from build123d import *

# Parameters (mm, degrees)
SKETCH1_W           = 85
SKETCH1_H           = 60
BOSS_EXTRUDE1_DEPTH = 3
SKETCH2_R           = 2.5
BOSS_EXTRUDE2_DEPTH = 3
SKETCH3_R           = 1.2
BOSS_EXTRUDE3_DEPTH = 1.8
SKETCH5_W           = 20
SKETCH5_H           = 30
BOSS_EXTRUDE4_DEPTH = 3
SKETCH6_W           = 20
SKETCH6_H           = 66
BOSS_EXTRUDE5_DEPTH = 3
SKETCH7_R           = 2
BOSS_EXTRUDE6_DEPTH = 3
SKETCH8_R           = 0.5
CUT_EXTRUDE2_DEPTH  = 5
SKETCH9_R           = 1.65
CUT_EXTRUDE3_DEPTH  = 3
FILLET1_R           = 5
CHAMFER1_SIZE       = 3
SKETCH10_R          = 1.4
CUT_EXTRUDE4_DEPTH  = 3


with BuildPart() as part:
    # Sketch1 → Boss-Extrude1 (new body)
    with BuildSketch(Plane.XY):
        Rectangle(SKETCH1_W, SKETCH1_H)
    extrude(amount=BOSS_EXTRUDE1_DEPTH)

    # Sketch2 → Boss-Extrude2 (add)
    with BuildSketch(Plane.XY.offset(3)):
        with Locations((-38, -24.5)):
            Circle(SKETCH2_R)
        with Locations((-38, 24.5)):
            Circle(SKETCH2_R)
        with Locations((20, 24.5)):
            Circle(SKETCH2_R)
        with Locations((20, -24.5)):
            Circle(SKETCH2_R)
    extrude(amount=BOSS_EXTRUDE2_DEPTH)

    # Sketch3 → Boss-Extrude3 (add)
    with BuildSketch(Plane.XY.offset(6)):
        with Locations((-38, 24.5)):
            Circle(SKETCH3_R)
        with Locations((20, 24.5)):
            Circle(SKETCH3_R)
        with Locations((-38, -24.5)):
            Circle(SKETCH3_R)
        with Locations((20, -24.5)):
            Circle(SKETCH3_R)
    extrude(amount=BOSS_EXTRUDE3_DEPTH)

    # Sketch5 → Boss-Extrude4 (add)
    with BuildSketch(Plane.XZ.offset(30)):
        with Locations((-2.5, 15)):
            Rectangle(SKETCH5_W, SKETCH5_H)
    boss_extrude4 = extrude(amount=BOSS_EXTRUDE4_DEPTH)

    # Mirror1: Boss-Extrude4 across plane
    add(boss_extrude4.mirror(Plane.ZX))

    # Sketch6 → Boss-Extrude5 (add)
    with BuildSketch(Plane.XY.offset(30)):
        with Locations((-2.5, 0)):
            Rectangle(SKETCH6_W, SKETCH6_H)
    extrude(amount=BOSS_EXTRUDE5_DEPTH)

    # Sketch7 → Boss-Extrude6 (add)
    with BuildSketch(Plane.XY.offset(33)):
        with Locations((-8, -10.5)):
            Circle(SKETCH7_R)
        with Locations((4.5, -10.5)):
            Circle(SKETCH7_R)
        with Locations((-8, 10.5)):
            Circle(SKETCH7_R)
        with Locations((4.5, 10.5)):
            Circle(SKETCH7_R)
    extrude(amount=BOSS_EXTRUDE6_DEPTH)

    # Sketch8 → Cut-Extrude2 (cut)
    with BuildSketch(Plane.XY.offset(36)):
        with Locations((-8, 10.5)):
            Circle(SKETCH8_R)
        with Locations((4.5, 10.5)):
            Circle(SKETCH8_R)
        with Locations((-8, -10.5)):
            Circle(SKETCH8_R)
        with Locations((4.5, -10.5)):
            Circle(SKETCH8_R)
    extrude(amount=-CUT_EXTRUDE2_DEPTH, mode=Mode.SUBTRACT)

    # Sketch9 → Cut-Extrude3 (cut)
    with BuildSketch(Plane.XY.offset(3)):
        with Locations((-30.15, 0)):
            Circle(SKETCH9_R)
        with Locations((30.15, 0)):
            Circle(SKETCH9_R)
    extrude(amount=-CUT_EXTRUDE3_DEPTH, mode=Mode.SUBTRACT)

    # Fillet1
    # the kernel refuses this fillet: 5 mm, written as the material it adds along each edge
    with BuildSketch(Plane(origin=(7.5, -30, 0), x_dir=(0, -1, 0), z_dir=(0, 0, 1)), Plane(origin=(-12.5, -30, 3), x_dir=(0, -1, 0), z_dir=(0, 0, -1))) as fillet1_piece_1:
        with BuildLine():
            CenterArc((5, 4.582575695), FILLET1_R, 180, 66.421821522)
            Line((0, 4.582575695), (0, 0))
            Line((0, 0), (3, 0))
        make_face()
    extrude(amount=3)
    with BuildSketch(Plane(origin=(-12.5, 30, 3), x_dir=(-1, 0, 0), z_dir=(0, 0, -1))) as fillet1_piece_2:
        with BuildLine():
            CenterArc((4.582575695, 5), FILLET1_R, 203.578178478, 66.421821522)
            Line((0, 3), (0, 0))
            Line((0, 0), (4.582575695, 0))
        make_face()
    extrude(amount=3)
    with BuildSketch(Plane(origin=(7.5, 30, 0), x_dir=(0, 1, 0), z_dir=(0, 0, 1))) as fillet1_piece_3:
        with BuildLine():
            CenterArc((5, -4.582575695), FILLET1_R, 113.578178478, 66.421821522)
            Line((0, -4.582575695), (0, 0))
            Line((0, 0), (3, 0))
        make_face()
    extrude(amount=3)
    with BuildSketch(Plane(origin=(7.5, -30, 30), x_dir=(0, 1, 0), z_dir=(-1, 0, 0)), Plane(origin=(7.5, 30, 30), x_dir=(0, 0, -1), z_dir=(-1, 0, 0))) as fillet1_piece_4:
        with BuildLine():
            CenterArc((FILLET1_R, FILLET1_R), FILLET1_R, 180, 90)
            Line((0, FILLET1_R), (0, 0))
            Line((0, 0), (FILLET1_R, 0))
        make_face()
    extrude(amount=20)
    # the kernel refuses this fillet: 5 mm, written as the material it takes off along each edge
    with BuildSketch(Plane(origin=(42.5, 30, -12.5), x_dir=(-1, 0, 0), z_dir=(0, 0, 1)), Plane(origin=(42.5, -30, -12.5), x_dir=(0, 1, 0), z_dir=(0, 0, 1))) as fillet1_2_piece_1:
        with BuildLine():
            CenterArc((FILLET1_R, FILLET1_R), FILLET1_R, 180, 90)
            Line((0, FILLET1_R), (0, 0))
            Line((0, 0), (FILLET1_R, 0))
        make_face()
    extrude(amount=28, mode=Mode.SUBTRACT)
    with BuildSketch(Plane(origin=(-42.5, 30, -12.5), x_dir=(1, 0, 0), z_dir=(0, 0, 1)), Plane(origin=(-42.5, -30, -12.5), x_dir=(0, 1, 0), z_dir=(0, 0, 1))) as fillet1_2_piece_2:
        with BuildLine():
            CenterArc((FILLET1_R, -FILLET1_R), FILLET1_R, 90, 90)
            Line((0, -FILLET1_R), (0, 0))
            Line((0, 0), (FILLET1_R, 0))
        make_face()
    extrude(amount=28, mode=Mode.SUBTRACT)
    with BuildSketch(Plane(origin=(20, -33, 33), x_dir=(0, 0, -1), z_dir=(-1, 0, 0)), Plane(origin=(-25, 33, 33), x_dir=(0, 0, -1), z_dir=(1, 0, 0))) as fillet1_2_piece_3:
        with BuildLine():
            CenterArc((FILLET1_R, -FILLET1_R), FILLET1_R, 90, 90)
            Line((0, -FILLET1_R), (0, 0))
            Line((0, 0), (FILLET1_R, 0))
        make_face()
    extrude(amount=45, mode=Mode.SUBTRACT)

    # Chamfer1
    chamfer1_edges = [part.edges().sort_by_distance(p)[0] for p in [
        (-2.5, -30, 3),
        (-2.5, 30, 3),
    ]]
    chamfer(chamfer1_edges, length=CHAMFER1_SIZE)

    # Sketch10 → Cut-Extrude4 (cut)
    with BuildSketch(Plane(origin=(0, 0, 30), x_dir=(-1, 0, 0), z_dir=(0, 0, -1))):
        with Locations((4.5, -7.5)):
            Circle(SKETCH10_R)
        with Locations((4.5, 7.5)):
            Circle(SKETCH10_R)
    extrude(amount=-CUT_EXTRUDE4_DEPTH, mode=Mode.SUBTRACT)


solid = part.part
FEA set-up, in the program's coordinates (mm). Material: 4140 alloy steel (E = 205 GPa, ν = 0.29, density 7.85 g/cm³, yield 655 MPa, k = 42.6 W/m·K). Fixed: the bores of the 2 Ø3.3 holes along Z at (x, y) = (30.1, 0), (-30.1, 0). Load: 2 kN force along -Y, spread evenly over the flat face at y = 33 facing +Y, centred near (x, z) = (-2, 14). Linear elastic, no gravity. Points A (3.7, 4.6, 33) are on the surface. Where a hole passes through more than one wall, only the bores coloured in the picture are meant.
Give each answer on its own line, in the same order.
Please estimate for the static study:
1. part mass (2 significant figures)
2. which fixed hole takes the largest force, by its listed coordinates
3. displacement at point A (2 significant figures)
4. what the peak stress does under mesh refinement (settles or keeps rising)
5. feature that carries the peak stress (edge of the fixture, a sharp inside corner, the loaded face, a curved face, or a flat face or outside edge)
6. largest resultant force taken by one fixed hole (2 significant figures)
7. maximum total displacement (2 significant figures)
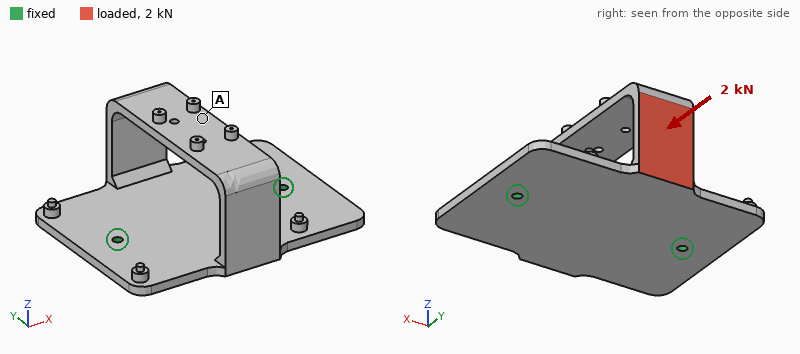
180 g
(-30.1, 0)
0.49 mm
keeps rising
edge of the fixture
1.1 kN
0.57 mm
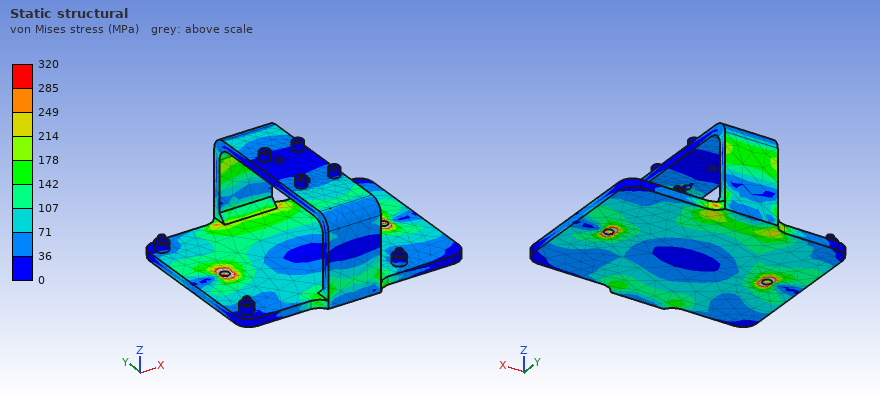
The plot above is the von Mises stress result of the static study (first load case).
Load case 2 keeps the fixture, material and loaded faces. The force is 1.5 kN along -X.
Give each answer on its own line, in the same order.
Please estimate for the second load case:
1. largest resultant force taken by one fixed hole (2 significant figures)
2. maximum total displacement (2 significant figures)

1.2 kN
0.25 mm
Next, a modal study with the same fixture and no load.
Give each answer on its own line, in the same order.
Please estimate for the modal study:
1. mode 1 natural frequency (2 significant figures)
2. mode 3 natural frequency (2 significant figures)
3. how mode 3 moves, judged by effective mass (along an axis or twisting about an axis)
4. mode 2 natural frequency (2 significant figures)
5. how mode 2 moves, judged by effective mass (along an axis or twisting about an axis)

810 Hz
1500 Hz
along X
1400 Hz
along Z
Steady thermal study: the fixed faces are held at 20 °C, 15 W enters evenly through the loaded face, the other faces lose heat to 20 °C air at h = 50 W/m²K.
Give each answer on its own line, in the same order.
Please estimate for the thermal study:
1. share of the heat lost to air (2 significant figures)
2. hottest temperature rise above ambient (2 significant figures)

73 %
63 K
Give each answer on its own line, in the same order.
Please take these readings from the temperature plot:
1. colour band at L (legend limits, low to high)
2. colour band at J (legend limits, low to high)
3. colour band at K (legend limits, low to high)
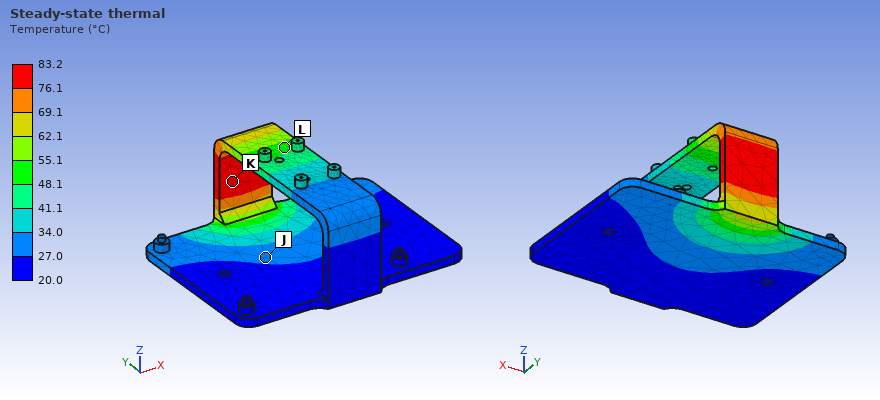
48.1 to 55.1 °C
27.0 to 34.0 °C
76.1 to 83.2 °C
